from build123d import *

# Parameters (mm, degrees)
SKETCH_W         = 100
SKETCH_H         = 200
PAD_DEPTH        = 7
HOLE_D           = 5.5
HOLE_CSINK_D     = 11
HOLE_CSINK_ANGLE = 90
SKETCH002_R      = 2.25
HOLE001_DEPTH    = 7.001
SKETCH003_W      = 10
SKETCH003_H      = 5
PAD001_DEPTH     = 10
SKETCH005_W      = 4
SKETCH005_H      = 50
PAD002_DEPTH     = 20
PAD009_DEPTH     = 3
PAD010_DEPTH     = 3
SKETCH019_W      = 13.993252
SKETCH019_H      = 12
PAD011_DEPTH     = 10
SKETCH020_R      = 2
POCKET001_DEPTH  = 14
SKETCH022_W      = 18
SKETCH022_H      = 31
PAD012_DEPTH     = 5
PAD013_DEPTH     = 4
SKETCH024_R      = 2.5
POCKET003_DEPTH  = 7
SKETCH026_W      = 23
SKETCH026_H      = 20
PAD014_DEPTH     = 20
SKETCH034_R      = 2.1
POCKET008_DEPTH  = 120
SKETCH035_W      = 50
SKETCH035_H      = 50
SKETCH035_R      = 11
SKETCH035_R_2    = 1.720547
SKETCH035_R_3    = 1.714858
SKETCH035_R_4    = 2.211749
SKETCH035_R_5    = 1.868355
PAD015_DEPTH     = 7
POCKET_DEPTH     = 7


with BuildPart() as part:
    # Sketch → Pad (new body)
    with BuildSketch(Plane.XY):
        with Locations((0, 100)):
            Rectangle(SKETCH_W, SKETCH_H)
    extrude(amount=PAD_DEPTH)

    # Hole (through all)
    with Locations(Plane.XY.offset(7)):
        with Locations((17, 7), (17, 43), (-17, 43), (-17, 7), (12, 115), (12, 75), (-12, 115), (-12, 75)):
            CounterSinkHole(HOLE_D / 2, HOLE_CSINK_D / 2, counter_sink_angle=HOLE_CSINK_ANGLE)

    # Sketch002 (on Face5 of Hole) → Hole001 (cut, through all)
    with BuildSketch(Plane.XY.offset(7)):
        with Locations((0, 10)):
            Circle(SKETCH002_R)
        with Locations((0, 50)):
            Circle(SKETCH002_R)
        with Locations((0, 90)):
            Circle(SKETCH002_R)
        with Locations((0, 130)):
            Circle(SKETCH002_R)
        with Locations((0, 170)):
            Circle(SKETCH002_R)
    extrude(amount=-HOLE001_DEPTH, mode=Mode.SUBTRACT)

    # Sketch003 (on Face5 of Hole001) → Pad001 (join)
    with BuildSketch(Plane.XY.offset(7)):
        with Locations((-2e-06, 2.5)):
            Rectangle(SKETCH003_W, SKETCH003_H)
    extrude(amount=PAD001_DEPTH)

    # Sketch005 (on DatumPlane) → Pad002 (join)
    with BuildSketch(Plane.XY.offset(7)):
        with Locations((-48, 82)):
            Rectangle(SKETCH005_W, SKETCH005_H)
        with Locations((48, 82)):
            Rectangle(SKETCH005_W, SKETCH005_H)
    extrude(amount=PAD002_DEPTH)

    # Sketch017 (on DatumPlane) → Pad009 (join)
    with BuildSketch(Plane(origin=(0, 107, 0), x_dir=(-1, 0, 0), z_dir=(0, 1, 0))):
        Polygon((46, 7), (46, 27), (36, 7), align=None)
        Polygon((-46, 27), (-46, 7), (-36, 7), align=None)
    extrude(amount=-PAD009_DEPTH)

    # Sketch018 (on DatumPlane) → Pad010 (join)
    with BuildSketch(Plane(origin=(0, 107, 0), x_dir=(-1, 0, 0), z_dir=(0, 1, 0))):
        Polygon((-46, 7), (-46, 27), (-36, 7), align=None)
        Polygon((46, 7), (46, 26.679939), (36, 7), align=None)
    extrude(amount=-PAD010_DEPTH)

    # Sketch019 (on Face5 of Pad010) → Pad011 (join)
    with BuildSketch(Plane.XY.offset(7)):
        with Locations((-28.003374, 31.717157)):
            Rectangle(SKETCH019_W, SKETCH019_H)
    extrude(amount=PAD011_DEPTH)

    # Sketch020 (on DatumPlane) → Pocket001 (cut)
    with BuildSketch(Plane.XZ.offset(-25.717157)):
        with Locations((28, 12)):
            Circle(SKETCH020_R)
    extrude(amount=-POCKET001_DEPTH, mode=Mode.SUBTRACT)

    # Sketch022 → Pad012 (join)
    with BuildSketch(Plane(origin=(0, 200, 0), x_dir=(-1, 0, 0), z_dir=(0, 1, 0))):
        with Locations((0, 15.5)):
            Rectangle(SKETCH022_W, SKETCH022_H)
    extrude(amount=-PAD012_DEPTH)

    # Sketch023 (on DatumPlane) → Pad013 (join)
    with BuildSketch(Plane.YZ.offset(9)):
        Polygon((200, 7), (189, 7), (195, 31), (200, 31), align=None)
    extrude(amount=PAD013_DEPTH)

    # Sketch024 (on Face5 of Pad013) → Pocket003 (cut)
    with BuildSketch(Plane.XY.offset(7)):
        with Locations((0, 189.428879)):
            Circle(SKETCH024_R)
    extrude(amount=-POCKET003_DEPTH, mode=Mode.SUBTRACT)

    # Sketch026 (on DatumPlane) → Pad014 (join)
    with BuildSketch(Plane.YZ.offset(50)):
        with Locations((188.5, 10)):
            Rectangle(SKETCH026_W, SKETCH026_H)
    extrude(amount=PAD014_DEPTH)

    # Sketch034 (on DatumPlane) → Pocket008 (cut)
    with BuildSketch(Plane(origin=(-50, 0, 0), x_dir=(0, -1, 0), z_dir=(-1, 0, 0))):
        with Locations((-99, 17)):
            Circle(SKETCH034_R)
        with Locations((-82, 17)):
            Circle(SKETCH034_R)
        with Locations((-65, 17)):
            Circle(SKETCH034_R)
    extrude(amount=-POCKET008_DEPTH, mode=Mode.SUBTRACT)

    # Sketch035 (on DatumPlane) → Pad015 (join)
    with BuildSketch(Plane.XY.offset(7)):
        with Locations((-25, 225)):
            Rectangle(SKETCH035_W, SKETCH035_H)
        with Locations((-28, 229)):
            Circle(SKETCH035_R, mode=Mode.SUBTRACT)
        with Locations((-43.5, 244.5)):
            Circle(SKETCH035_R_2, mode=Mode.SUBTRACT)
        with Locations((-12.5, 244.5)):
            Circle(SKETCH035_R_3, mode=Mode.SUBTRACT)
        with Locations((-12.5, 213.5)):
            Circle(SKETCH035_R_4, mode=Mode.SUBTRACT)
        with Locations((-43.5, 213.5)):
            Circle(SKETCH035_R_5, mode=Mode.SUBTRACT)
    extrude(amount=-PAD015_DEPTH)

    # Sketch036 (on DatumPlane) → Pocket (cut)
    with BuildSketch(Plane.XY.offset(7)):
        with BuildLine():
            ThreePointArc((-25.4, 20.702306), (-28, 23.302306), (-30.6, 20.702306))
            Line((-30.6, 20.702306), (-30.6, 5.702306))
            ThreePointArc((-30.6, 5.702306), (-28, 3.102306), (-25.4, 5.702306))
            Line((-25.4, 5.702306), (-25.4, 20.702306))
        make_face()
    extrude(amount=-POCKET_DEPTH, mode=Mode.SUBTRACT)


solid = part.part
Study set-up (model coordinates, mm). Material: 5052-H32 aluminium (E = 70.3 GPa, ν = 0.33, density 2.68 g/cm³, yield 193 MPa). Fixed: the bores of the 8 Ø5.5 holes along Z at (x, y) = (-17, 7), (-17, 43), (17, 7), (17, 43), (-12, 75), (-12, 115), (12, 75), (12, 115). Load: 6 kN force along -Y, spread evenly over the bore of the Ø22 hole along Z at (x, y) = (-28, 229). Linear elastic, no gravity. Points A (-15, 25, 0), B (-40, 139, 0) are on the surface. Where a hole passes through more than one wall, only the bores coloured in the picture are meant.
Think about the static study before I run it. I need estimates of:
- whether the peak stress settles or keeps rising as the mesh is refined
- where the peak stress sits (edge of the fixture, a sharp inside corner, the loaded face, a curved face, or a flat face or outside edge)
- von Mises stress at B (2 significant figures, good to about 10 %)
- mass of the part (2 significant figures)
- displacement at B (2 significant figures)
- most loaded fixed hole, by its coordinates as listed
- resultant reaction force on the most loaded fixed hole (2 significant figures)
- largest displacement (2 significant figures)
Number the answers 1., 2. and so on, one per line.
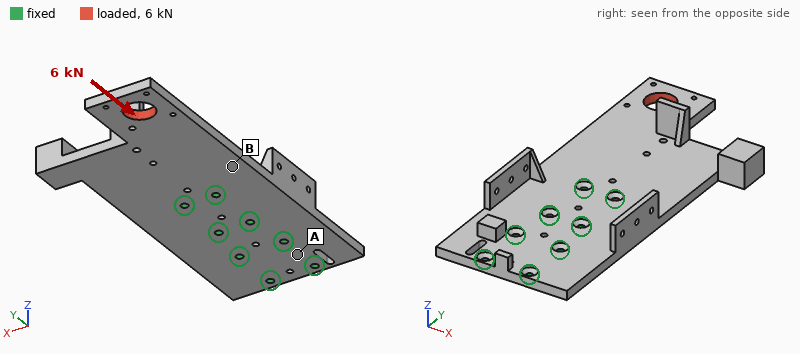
1. keeps rising
2. edge of the fixture
3. 18 MPa
4. 470 g
5. 18 µm
6. (-12, 115)
7. 3.6 kN
8. 83 µm
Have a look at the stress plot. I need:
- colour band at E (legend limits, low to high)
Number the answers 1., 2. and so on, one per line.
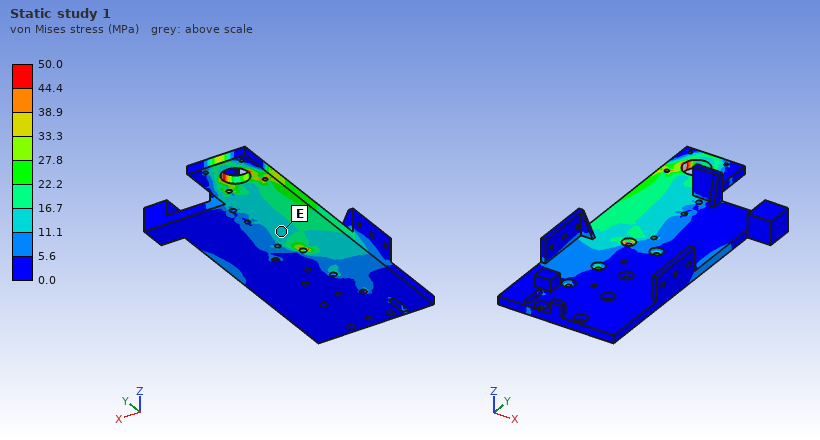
1. 11.1 to 16.7 MPa
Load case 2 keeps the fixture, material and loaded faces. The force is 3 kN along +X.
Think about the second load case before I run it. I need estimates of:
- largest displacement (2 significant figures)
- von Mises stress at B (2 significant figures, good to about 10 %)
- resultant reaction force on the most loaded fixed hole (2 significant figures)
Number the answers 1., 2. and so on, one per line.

1. 0.19 mm
2. 20 MPa
3. 4.2 kN
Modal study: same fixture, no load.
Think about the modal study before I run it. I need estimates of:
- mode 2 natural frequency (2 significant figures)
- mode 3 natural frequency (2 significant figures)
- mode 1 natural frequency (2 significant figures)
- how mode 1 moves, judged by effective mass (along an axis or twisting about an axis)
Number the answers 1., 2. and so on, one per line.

1. 730 Hz
2. 1800 Hz
3. 380 Hz
4. along Z
